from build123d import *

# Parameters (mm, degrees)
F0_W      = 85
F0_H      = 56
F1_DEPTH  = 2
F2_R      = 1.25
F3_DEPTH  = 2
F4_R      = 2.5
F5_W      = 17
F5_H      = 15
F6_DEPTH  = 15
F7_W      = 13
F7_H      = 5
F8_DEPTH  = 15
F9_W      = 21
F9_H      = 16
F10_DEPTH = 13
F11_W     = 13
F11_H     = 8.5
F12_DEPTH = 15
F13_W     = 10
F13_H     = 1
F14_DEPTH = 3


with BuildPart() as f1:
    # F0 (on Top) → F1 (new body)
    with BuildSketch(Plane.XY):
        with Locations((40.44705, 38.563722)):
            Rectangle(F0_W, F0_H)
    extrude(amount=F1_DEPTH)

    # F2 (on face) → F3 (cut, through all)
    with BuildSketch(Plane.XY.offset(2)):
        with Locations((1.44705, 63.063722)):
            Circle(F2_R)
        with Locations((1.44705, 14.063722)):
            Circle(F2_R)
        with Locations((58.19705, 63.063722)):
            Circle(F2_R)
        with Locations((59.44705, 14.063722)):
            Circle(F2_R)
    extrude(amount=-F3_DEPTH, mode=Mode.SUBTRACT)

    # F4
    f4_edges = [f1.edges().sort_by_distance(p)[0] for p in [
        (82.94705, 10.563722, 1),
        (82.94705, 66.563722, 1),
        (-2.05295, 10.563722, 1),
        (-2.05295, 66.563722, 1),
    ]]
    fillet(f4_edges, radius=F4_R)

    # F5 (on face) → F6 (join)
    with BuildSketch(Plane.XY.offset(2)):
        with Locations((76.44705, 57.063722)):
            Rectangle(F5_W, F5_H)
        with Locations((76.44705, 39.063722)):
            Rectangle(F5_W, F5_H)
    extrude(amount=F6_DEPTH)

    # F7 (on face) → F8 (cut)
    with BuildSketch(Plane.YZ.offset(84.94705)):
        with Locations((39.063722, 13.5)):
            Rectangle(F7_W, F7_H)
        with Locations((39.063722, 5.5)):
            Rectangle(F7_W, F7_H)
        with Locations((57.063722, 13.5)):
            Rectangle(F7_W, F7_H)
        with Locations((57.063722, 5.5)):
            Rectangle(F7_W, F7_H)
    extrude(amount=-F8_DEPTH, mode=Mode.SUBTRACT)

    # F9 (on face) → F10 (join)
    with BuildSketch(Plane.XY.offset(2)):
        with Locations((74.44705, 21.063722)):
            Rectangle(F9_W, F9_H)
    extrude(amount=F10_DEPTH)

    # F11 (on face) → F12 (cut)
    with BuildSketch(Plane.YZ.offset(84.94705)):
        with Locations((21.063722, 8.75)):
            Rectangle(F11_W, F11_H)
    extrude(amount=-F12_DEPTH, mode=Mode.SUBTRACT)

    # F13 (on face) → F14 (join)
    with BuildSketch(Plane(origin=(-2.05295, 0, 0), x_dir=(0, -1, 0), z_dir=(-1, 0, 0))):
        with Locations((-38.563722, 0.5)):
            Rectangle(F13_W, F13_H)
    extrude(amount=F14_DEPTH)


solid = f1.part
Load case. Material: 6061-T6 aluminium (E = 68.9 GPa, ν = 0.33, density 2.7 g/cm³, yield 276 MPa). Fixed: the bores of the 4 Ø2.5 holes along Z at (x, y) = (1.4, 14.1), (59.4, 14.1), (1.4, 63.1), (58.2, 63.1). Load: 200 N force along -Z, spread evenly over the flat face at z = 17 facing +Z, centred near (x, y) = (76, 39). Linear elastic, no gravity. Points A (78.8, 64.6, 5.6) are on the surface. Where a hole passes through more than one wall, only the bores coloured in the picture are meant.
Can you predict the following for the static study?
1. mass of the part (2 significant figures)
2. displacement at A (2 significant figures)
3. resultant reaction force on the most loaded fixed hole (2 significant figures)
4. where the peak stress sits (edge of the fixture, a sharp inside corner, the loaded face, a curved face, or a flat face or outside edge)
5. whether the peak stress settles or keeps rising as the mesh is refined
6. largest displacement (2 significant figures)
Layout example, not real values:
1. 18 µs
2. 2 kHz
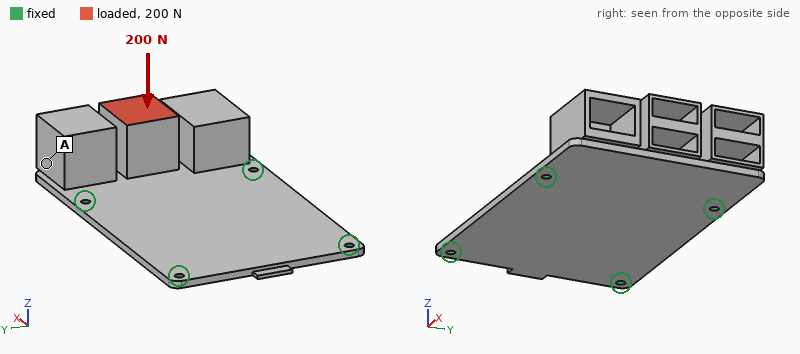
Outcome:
1. 43 g
2. 0.22 mm
3. 110 N
4. edge of the fixture
5. keeps rising
6. 0.44 mm
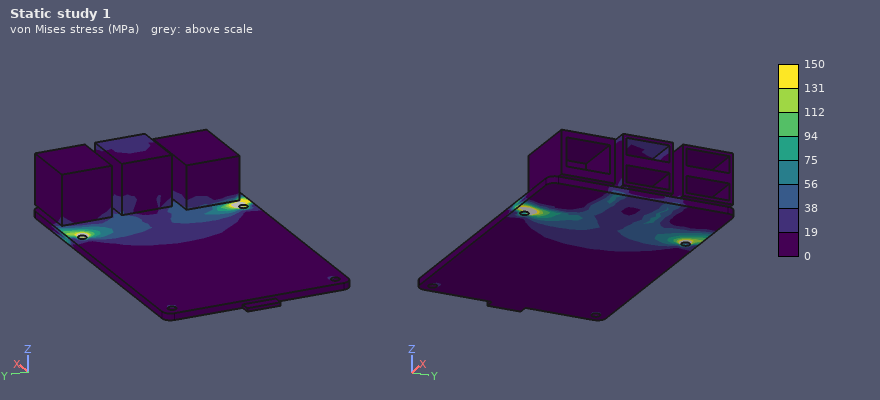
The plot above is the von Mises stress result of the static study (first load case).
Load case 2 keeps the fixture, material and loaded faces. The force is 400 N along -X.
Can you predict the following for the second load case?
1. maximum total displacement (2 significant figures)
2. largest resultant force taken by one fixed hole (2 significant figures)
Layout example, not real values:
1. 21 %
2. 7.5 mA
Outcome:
1. 0.81 mm
2. 160 N
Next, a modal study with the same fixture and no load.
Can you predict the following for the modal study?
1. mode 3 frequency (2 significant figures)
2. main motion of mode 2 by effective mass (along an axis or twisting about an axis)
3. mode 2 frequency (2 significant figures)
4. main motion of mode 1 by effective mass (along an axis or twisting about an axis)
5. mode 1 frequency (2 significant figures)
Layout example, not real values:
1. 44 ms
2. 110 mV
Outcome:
1. 3100 Hz
2. along Z
3. 2300 Hz
4. along Z
5. 980 Hz
